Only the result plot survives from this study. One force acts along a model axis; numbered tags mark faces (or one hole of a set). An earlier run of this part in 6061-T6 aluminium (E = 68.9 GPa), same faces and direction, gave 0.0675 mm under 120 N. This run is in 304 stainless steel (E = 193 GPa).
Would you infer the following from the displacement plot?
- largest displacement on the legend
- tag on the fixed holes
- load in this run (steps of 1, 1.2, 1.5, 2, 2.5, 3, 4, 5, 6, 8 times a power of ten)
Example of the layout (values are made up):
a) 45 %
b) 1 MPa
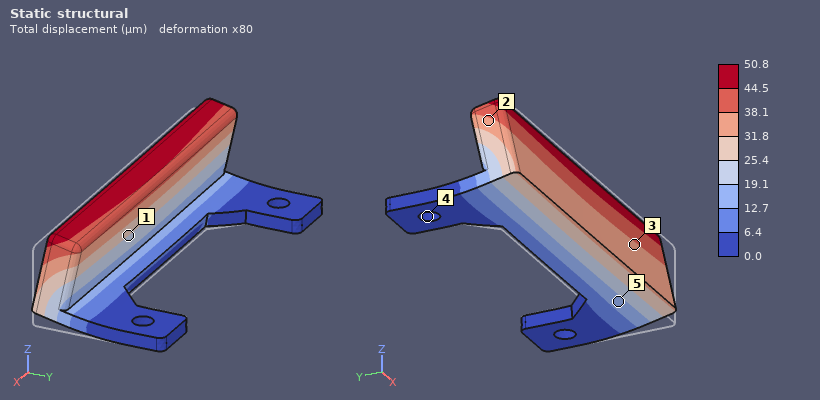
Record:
a) 50.8 µm
b) 4
c) 250 N
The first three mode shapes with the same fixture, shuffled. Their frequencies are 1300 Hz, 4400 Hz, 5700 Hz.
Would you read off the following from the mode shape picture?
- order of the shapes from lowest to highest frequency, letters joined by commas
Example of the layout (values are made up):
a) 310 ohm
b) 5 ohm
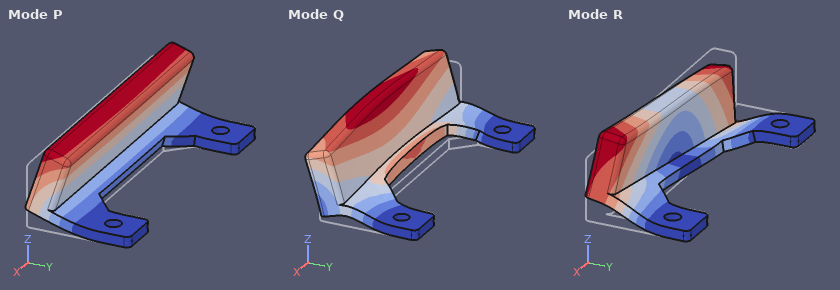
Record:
a) P, R, Q
